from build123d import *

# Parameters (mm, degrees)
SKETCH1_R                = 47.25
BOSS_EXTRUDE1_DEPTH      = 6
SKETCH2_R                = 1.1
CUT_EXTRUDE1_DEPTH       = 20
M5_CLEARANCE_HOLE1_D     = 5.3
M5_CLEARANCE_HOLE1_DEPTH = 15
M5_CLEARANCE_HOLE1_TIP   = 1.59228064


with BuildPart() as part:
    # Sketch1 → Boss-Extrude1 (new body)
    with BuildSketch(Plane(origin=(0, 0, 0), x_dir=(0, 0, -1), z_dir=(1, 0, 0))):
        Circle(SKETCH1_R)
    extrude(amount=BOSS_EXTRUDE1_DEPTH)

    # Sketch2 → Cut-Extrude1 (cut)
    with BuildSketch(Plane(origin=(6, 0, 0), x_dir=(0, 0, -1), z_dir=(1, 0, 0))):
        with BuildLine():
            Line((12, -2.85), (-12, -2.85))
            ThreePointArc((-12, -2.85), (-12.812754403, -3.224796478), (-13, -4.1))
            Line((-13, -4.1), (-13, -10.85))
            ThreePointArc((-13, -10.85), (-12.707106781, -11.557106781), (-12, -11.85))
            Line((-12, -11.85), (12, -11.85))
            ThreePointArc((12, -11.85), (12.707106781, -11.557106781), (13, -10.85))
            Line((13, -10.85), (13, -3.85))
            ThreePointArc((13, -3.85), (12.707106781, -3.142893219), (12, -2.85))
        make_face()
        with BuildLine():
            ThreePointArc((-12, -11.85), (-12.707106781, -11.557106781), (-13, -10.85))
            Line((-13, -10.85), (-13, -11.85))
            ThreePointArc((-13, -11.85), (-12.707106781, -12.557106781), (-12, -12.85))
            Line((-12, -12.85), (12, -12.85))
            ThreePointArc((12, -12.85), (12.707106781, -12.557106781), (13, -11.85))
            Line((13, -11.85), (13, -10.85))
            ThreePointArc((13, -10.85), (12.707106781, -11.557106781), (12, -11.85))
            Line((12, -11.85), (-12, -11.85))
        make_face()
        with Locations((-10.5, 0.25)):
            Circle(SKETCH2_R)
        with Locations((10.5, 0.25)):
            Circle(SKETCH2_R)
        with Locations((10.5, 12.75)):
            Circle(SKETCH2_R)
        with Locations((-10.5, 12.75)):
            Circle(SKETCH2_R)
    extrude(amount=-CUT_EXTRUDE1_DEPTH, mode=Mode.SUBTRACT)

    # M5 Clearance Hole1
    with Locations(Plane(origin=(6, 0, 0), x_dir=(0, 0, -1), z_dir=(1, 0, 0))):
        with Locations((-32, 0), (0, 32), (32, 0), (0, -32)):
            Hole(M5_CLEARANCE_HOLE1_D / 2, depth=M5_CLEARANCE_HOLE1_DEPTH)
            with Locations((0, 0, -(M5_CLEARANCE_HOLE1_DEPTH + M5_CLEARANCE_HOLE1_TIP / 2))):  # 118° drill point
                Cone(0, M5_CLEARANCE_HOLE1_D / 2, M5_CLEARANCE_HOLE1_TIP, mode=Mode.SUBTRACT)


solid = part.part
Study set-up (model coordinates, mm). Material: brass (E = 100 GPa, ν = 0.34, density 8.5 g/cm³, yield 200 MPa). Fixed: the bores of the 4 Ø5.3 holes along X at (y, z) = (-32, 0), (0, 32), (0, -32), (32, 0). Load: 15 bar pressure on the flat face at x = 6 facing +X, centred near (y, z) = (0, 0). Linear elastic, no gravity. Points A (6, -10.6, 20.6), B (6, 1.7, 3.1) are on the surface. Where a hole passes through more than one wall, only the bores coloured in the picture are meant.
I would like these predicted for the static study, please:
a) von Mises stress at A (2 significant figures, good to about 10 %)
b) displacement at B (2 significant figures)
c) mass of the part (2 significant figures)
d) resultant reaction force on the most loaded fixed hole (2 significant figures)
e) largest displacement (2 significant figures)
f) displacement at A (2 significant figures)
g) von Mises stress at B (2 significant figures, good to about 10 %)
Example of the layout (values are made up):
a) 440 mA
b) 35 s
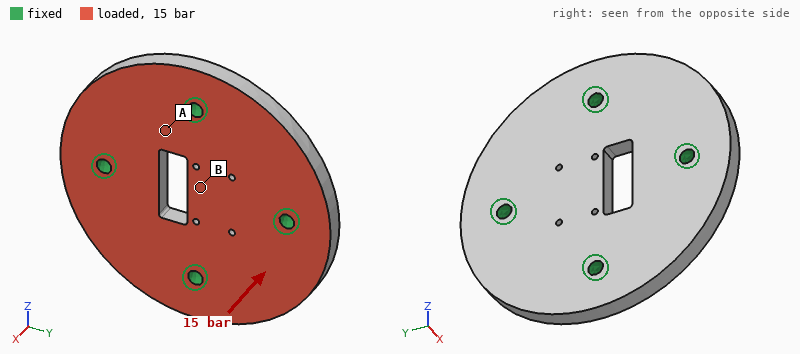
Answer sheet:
a) 28 MPa
b) 16 µm
c) 340 g
d) 2.5 kN
e) 38 µm
f) 10 µm
g) 13 MPa
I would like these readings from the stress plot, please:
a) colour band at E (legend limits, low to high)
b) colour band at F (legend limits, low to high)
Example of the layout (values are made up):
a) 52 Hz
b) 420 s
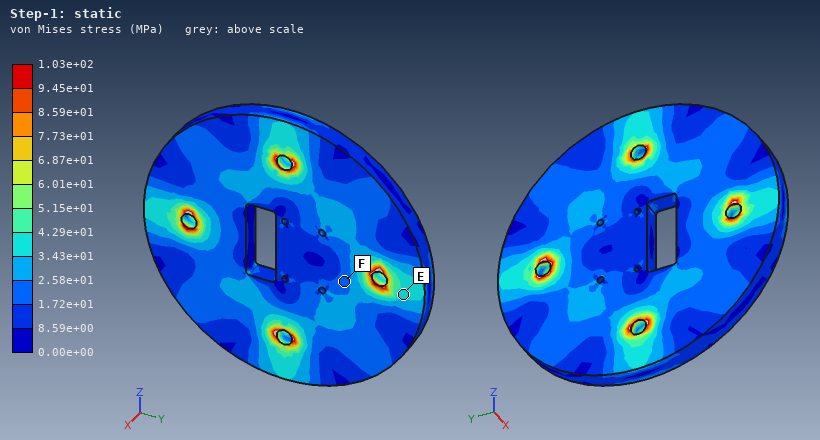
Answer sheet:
a) 3.43e+01 to 4.29e+01 MPa
b) 1.72e+01 to 2.58e+01 MPa
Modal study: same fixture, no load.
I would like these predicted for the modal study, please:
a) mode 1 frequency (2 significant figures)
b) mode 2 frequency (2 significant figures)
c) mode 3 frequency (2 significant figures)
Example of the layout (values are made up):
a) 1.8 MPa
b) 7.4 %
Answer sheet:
a) 4800 Hz
b) 5300 Hz
c) 5300 Hz
